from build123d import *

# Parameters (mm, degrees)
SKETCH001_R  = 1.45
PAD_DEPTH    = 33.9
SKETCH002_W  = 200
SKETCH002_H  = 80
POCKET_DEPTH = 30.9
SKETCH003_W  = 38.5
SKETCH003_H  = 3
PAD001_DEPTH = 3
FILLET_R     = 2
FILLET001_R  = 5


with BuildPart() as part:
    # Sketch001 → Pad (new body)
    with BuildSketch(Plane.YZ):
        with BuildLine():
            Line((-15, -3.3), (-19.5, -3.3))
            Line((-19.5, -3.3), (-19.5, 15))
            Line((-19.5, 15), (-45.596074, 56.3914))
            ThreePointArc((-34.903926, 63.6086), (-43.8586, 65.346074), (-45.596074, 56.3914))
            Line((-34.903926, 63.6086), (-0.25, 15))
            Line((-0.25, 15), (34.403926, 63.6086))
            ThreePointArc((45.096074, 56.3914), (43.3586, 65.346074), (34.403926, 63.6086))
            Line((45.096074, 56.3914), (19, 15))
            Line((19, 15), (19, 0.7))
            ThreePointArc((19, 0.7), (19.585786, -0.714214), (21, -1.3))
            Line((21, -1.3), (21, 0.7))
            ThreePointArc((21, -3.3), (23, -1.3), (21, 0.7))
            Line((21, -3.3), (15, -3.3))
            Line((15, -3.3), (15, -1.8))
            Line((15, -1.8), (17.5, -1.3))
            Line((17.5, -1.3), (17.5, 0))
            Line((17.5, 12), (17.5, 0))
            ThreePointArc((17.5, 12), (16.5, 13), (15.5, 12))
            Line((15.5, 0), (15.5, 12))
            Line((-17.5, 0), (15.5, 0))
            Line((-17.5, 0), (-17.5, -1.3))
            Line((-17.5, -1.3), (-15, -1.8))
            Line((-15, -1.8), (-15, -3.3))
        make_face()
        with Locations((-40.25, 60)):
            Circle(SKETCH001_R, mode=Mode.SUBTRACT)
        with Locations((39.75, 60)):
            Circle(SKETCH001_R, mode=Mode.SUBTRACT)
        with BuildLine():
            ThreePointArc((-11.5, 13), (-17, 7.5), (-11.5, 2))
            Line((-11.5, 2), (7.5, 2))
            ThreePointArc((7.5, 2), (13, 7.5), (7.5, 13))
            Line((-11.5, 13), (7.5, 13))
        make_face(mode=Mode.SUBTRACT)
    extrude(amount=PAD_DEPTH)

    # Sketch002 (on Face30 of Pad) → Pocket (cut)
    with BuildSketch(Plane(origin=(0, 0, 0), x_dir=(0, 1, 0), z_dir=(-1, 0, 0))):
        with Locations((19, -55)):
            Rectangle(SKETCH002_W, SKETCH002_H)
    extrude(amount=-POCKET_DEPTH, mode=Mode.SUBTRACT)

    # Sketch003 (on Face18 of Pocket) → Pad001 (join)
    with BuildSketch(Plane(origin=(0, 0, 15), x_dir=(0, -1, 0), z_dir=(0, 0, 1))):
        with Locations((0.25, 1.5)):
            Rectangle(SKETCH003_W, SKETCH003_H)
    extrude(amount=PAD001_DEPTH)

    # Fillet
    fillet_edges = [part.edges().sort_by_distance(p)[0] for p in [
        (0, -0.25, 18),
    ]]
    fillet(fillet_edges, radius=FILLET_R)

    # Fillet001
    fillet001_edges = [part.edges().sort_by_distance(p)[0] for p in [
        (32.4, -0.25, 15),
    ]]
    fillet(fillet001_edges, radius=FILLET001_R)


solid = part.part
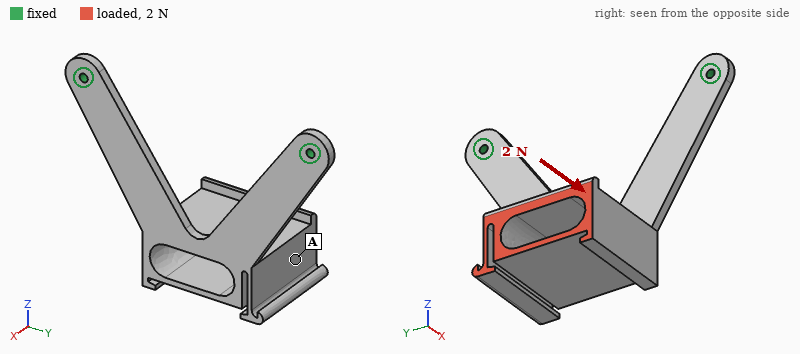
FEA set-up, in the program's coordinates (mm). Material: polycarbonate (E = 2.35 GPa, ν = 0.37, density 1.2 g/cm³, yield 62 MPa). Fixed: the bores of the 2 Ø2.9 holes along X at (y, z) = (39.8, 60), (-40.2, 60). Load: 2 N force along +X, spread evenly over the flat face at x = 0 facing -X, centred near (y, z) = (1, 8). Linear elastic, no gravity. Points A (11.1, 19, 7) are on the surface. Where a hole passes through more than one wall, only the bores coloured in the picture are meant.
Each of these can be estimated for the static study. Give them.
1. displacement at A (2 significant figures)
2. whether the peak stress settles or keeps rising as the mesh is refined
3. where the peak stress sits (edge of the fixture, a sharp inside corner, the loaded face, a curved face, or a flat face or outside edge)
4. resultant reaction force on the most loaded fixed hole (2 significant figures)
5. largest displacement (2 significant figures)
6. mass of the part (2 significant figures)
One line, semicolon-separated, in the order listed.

0.89 mm; keeps rising; edge of the fixture; 1.0 N; 1.2 mm; 18 g
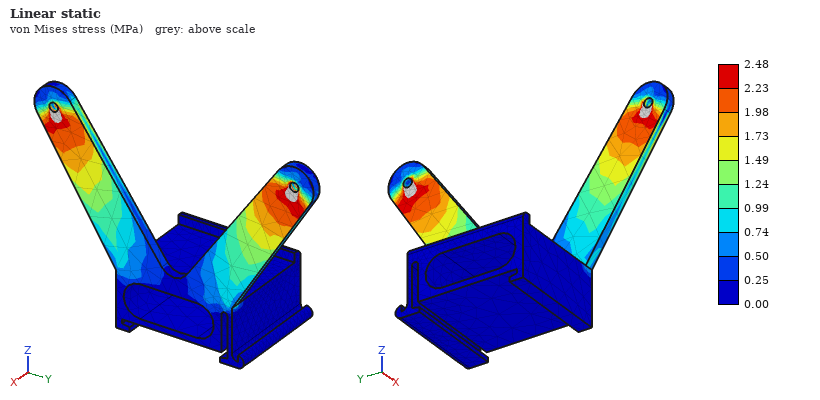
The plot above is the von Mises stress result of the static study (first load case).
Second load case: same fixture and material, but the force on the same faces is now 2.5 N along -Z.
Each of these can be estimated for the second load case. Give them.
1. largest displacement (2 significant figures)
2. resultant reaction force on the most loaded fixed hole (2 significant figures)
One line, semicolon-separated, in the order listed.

1.4 mm; 1.6 N
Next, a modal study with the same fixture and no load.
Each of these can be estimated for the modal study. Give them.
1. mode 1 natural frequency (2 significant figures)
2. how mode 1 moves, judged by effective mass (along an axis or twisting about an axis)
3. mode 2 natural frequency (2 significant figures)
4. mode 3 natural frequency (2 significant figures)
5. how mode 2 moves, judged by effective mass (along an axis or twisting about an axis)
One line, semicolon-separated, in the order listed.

63 Hz; along X; 210 Hz; 280 Hz; along Y
